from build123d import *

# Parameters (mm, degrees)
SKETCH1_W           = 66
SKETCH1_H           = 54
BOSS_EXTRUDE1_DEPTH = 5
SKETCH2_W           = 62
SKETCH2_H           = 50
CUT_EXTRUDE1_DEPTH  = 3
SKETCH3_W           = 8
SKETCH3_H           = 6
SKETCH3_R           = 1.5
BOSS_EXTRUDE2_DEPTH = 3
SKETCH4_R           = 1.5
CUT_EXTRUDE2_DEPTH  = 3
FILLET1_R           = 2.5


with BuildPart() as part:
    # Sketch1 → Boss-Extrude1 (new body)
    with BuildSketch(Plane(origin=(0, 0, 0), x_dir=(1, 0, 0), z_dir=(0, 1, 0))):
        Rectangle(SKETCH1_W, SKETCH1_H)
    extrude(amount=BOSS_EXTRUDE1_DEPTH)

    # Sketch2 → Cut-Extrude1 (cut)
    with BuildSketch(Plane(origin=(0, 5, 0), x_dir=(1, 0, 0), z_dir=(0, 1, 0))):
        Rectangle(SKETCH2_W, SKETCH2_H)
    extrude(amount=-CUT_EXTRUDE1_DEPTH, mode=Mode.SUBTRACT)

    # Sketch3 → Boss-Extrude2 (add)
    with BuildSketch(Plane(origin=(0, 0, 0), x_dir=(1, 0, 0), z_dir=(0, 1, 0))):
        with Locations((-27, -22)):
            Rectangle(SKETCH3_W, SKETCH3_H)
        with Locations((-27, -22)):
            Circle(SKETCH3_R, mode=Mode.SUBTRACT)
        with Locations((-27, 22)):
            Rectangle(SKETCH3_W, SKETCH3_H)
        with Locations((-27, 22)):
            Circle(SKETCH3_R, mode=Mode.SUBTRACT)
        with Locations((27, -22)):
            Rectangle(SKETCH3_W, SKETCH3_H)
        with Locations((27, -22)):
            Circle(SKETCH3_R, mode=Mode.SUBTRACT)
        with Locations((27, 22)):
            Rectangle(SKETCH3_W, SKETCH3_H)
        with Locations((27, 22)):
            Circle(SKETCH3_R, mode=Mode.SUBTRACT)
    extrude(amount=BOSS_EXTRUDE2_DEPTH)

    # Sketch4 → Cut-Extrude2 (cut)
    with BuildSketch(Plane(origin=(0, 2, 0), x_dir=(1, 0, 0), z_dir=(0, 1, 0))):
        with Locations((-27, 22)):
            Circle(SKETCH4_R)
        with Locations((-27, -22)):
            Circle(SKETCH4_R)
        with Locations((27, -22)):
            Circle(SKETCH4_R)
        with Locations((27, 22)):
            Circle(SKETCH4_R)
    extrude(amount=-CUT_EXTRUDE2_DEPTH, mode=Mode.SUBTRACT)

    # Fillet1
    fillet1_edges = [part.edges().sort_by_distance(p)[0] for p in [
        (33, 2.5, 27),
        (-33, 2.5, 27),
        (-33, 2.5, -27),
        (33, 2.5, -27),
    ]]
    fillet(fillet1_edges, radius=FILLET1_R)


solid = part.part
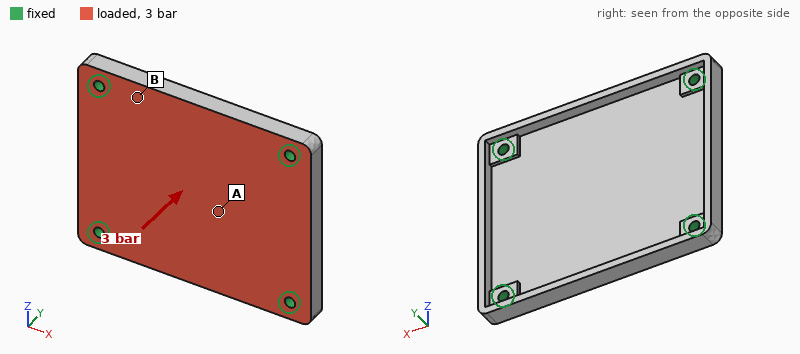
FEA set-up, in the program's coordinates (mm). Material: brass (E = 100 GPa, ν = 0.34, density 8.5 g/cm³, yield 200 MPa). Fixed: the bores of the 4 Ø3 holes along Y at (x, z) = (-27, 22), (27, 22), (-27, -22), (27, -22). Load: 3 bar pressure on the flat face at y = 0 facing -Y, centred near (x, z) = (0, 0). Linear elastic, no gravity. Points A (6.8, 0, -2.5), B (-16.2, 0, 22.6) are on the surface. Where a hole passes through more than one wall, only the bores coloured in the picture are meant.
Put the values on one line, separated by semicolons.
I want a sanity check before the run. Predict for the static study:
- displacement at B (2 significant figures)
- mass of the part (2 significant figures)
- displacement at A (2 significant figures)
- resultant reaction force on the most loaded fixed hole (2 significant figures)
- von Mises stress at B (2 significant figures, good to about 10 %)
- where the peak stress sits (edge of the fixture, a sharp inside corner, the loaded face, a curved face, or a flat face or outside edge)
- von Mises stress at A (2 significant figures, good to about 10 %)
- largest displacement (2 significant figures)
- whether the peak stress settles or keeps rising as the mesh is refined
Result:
0.020 mm; 73 g; 0.10 mm; 280 N; 29 MPa; edge of the fixture; 47 MPa; 0.11 mm; keeps rising
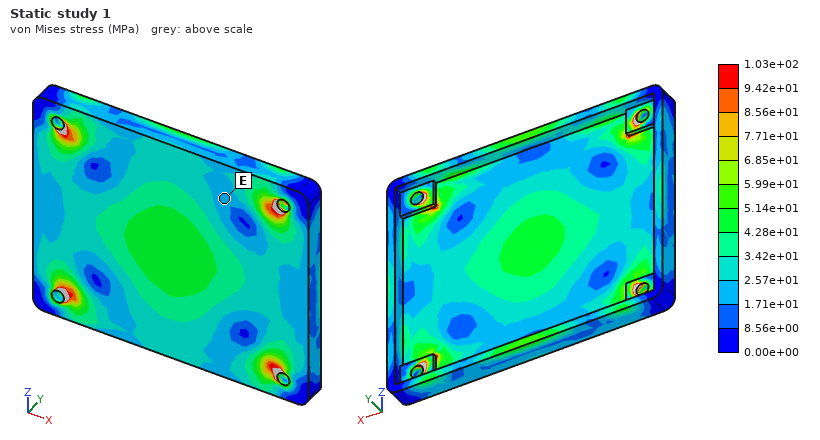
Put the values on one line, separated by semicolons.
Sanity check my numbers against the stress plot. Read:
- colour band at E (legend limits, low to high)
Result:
1.71e+01 to 2.57e+01 MPa
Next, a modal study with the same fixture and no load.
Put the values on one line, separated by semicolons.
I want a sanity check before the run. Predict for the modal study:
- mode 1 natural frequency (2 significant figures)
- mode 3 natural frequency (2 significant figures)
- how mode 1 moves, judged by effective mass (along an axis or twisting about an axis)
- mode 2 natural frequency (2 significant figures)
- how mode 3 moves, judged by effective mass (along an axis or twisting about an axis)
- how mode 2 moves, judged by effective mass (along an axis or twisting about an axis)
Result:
2500 Hz; 5000 Hz; along Y; 4400 Hz; twisting about Z; twisting about X
